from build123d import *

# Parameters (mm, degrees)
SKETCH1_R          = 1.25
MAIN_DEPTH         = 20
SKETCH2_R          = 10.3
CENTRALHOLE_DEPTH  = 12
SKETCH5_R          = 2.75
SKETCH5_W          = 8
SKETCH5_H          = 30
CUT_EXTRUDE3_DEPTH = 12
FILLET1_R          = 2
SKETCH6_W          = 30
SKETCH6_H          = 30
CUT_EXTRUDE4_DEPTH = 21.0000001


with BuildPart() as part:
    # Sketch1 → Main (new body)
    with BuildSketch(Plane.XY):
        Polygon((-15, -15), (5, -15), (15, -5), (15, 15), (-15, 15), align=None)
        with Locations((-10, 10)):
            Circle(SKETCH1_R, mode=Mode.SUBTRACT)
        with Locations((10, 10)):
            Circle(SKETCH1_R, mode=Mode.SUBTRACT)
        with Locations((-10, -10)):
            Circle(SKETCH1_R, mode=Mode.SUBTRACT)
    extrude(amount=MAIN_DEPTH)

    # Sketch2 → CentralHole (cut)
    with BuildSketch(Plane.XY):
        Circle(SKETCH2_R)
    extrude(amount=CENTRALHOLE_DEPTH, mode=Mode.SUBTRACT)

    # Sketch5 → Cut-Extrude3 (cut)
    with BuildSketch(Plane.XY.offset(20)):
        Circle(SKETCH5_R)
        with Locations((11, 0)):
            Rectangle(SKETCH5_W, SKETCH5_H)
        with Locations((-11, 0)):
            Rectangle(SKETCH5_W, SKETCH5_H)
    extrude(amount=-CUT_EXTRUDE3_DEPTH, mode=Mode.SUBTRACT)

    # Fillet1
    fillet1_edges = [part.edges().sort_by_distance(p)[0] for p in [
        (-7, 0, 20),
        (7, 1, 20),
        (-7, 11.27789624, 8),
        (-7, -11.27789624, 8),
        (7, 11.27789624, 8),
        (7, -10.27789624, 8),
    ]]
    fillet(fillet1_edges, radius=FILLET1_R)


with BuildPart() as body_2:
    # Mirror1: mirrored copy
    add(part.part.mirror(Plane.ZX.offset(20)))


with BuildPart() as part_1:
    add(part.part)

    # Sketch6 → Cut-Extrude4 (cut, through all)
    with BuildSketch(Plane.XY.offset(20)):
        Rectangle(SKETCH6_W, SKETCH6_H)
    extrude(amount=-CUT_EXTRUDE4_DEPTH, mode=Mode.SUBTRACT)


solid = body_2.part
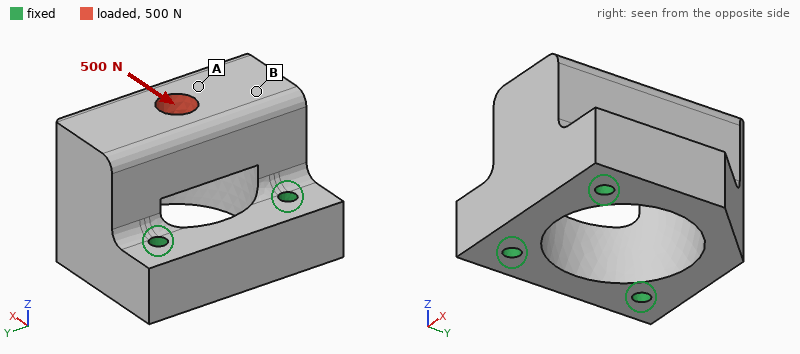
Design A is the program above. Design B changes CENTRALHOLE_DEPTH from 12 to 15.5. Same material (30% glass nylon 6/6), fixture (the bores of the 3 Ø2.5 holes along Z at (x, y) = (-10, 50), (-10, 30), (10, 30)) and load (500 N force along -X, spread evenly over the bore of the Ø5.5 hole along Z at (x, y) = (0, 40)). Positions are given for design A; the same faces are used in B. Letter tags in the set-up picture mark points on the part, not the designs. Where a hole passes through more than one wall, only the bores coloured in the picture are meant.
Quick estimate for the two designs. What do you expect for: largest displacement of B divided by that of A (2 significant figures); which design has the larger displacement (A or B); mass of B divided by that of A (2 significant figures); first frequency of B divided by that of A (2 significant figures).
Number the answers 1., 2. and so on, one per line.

1. 1.4
2. B
3. 0.89
4. 0.99
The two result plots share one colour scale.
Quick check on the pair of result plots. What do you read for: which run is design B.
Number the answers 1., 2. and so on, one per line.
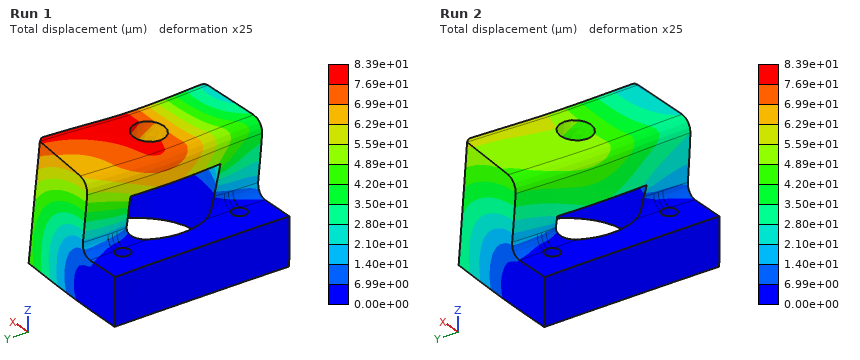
1. Run 1
